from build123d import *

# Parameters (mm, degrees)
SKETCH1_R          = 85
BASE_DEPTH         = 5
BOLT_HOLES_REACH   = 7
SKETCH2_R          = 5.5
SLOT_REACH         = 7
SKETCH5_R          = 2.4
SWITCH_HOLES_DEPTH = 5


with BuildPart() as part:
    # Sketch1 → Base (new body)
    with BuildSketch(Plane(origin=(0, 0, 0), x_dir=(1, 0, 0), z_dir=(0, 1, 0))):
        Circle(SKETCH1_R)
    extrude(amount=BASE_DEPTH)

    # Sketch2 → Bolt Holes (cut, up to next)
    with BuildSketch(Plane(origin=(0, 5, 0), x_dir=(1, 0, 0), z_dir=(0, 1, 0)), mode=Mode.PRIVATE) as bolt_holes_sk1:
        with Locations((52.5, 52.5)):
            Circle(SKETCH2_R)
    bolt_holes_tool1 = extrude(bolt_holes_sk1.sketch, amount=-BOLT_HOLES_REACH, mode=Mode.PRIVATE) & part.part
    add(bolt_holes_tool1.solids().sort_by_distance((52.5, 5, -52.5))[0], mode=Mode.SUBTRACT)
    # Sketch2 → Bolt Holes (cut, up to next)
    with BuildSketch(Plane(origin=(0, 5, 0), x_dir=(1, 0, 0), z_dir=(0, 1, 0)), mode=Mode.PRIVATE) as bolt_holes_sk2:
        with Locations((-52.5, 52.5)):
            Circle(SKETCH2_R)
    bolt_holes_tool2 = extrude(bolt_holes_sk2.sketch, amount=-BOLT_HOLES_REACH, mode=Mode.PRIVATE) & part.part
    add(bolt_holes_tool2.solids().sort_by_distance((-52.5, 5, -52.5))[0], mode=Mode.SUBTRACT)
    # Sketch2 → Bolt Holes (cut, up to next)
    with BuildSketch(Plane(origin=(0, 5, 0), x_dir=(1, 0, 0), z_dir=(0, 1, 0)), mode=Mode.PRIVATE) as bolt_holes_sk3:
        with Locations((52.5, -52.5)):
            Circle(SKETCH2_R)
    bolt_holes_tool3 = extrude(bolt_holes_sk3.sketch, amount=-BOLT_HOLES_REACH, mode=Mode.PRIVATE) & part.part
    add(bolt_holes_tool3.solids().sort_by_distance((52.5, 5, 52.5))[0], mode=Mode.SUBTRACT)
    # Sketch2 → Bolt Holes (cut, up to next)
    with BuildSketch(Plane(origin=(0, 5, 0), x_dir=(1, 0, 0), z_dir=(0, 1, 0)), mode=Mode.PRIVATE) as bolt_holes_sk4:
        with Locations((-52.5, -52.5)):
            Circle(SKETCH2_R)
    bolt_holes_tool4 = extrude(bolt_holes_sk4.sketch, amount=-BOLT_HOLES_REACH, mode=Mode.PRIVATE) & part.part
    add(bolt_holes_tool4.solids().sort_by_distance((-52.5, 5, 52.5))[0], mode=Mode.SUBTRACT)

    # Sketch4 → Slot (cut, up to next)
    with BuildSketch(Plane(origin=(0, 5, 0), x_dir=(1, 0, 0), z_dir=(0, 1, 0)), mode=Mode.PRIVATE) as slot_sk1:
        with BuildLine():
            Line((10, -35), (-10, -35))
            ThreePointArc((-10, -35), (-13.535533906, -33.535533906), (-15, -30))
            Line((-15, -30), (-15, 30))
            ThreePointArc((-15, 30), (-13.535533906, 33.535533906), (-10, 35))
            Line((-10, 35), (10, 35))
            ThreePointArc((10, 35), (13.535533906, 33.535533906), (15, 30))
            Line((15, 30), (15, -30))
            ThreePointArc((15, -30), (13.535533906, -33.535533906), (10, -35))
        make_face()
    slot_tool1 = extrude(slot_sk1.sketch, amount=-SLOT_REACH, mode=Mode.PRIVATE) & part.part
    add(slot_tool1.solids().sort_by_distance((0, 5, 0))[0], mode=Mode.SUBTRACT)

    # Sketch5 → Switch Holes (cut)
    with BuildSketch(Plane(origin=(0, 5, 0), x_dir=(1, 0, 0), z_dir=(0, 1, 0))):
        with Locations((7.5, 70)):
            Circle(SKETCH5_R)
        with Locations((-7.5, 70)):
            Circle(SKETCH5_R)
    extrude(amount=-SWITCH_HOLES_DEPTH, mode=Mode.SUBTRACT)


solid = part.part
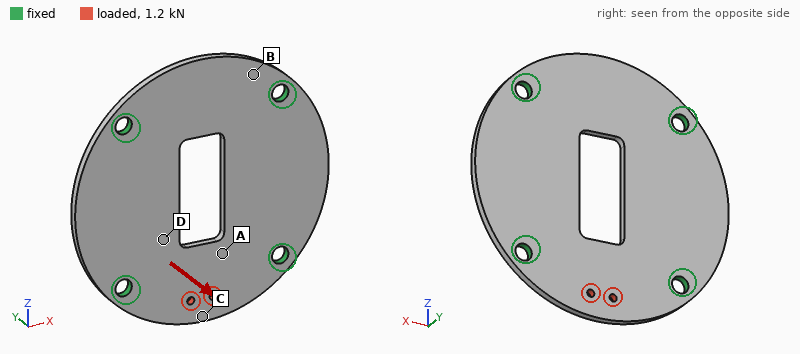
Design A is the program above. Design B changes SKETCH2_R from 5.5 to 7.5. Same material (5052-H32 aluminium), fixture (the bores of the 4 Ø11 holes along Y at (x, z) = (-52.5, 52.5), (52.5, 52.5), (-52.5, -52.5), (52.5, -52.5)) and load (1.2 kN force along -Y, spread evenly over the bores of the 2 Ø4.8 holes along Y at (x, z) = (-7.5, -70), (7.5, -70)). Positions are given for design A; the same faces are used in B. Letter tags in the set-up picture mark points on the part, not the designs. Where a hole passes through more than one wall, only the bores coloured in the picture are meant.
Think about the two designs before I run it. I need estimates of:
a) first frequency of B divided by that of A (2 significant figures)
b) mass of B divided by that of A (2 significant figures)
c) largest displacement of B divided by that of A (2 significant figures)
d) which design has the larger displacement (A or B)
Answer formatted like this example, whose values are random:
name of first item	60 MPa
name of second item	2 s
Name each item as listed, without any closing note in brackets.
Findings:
first frequency of B divided by that of A	1.1
mass of B divided by that of A	0.98
largest displacement of B divided by that of A	0.88
which design has the larger displacement	A
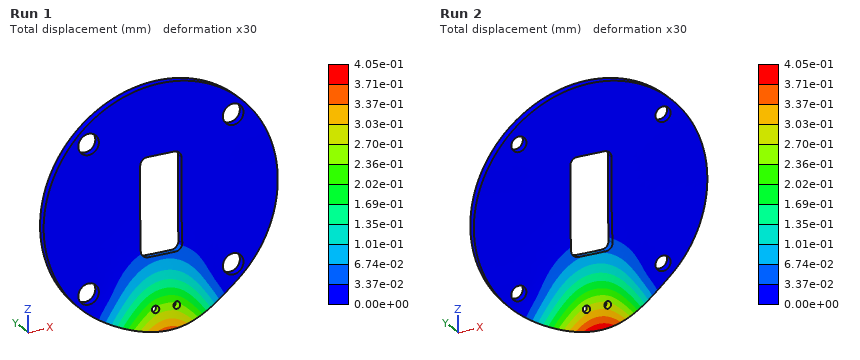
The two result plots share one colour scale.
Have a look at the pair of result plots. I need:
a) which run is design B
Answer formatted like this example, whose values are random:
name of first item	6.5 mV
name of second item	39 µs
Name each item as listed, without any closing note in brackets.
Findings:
which run is design B	Run 1
